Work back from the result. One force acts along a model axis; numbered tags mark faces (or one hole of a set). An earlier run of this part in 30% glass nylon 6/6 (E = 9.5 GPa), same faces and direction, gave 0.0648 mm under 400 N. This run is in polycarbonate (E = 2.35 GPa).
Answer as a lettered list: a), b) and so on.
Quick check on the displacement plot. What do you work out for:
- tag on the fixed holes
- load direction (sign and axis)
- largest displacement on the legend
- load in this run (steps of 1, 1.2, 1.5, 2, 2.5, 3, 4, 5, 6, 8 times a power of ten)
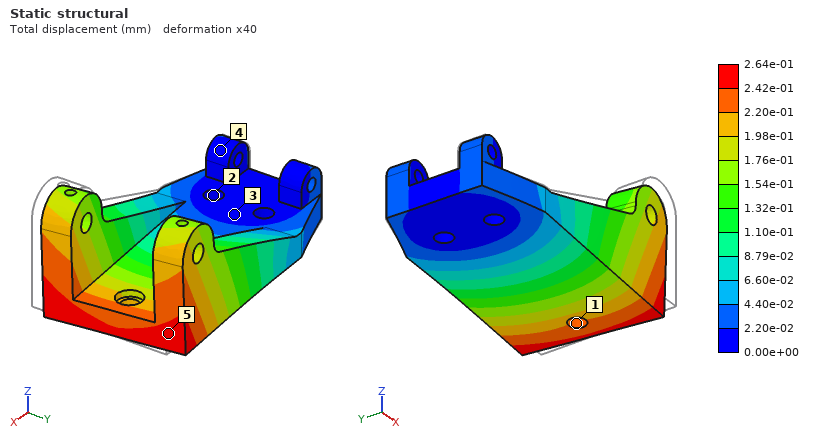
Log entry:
a) 2
b) +Y
c) 2.64e-01 mm
d) 400 N
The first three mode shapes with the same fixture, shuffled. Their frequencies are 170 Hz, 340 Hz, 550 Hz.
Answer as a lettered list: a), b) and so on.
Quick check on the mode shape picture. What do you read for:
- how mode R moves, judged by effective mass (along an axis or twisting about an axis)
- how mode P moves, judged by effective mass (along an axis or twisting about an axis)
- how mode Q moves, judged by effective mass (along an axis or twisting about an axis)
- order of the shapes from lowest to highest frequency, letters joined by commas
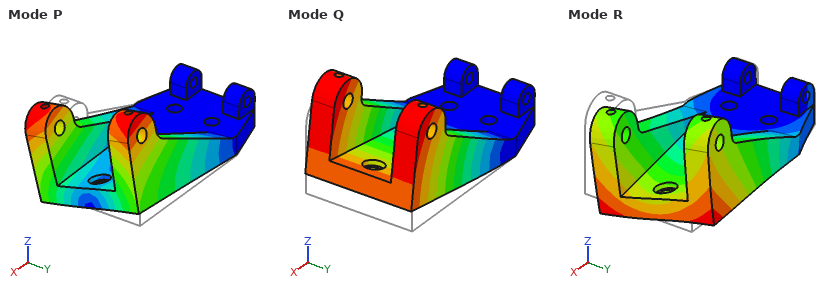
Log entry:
a) along Y
b) along Y
c) along Z
d) Q, P, R
